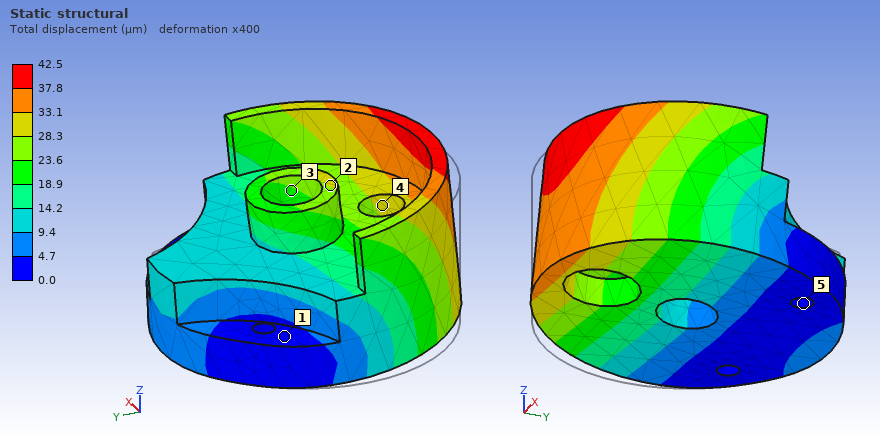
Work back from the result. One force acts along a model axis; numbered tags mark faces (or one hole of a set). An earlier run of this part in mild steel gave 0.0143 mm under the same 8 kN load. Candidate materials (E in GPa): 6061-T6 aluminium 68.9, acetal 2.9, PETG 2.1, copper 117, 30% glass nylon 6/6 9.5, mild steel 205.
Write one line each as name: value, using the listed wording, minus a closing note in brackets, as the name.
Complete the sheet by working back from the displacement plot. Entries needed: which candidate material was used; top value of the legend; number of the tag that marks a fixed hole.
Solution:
which candidate material was used: 6061-T6 aluminium
top value of the legend: 42.5 µm
number of the tag that marks a fixed hole: 5
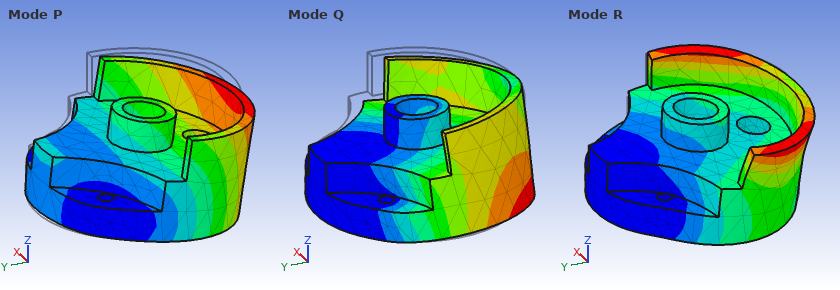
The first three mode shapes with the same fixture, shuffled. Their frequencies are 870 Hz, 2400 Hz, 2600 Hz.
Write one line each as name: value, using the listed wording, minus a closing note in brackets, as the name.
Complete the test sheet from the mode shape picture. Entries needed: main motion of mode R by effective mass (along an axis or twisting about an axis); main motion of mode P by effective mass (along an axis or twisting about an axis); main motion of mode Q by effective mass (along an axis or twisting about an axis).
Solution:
main motion of mode R by effective mass: along X
main motion of mode P by effective mass: along Z
main motion of mode Q by effective mass: along X
